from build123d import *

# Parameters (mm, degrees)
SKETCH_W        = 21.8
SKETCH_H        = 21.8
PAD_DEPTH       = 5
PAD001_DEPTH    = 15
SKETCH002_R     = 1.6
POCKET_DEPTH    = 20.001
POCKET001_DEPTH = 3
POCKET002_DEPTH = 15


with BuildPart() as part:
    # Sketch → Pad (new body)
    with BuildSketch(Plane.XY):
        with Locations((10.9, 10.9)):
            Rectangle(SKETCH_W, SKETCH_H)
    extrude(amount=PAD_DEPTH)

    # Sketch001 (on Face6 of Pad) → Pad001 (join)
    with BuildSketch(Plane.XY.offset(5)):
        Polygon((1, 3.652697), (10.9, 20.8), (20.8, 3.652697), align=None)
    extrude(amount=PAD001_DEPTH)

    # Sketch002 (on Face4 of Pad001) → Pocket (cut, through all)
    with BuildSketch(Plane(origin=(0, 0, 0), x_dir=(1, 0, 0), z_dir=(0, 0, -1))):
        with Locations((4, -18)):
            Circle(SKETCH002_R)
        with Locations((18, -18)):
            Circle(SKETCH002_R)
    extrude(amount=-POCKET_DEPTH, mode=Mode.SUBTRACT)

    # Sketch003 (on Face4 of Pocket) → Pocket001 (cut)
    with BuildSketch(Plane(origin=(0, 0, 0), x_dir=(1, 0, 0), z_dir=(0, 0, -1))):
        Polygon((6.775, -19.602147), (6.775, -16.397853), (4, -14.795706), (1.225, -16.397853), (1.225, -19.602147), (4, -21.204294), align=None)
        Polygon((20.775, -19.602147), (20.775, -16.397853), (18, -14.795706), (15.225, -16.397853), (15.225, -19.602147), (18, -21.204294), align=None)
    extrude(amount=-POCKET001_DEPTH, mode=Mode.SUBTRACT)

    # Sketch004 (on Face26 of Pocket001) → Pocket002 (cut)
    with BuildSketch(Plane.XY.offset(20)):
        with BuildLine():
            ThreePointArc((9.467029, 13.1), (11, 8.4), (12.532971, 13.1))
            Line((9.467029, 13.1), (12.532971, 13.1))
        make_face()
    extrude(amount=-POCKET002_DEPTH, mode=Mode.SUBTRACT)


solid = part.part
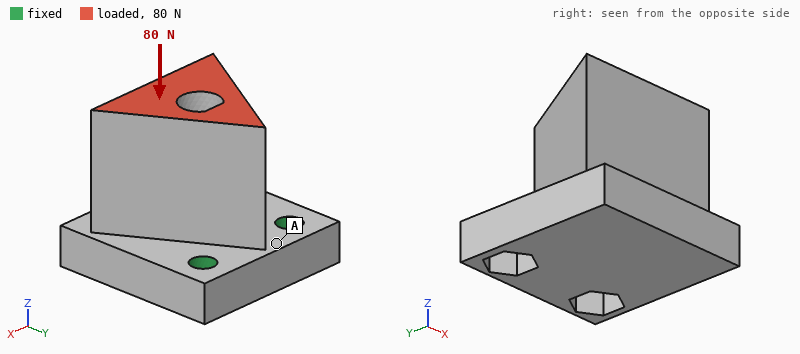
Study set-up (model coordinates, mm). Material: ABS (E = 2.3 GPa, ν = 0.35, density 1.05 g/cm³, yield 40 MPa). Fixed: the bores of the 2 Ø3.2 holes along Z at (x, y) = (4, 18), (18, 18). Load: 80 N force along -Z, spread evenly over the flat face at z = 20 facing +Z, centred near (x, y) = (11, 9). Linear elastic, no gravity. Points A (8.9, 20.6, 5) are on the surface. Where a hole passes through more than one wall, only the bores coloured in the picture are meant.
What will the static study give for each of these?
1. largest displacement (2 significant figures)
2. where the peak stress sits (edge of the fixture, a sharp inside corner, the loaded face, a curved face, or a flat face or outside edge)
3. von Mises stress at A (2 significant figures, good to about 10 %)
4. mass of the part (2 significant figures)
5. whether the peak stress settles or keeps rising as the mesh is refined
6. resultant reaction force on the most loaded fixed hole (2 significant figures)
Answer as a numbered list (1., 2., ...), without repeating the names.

1. 0.36 mm
2. edge of the fixture
3. 3.7 MPa
4. 4.6 g
5. keeps rising
6. 41 N
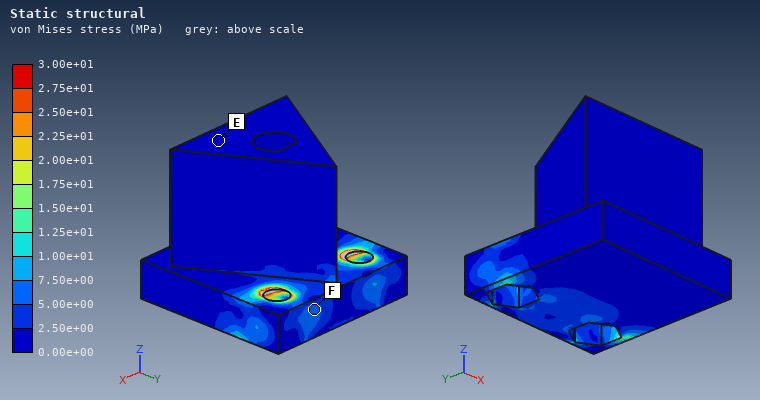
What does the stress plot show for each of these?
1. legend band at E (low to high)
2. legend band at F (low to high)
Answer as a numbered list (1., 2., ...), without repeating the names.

1. 0.00e+00 to 2.50e+00 MPa
2. 5.00e+00 to 7.50e+00 MPa
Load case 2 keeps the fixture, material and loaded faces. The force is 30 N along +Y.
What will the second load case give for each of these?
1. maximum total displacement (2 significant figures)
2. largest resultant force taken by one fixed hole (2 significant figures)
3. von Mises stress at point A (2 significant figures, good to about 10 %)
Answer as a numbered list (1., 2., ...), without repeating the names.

1. 0.28 mm
2. 16 N
3. 3.7 MPa
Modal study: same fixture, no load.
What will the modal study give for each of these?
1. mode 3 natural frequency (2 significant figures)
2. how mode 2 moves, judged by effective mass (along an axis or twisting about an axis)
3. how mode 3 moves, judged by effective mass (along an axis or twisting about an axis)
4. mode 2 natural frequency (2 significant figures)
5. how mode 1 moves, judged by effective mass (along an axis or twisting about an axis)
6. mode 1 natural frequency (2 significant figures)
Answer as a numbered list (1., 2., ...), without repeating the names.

1. 6200 Hz
2. along X
3. along X
4. 2900 Hz
5. along Z
6. 1200 Hz
